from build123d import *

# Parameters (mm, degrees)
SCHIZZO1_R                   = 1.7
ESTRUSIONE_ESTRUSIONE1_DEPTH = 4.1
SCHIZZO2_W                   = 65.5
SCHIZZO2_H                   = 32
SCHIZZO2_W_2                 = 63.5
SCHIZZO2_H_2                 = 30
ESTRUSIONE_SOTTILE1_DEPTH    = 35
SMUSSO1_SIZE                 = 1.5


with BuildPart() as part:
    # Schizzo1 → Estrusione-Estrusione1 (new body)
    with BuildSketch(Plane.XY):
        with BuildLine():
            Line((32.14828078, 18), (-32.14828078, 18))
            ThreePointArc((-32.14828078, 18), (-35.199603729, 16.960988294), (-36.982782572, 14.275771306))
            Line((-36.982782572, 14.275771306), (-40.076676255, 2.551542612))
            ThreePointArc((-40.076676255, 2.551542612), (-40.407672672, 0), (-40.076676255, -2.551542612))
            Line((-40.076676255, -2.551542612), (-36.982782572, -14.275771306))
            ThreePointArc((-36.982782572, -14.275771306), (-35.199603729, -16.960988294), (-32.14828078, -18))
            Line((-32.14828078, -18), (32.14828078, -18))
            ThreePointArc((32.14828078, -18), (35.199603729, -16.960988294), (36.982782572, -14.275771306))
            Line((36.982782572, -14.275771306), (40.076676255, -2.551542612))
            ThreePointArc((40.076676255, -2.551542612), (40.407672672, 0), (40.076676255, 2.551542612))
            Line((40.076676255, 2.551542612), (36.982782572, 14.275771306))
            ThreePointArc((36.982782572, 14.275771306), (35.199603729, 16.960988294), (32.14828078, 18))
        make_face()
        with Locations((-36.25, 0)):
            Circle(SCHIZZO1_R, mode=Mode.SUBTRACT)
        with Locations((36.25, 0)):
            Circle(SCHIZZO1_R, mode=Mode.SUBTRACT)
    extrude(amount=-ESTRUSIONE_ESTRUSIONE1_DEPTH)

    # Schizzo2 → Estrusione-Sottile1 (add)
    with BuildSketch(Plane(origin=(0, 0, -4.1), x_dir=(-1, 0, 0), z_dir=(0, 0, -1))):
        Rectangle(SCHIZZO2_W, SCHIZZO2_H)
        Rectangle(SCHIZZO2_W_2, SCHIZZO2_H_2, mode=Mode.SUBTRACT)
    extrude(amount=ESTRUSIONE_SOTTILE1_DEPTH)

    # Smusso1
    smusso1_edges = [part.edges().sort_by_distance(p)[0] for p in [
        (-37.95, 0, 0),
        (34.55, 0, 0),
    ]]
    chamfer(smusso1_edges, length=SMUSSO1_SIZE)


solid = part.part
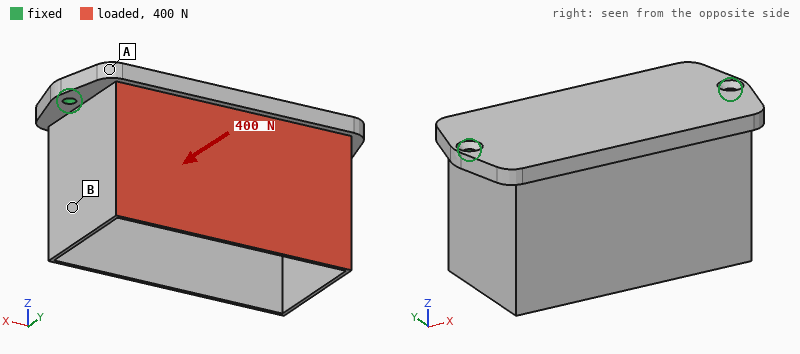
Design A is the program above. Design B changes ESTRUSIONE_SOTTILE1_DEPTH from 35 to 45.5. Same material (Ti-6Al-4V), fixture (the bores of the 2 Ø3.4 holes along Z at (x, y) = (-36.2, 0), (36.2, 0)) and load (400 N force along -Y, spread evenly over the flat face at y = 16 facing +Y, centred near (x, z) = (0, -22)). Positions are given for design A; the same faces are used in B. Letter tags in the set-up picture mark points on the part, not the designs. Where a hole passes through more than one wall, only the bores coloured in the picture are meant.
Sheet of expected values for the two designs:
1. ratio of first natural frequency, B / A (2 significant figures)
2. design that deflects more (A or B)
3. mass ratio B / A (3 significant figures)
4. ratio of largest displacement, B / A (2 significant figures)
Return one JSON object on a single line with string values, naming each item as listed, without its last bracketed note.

{"ratio of first natural frequency, B / A": "0.81", "design that deflects more": "B", "mass ratio B / A": "1.11", "ratio of largest displacement, B / A": "1.1"}
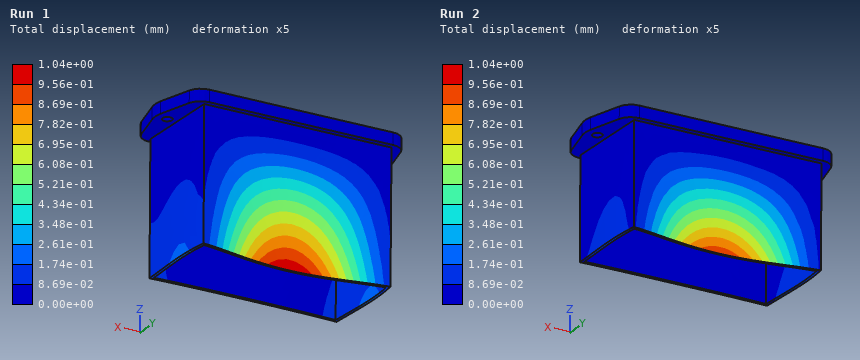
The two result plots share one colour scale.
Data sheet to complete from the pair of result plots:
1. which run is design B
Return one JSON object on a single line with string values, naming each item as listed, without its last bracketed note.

{"which run is design B": "Run 1"}
